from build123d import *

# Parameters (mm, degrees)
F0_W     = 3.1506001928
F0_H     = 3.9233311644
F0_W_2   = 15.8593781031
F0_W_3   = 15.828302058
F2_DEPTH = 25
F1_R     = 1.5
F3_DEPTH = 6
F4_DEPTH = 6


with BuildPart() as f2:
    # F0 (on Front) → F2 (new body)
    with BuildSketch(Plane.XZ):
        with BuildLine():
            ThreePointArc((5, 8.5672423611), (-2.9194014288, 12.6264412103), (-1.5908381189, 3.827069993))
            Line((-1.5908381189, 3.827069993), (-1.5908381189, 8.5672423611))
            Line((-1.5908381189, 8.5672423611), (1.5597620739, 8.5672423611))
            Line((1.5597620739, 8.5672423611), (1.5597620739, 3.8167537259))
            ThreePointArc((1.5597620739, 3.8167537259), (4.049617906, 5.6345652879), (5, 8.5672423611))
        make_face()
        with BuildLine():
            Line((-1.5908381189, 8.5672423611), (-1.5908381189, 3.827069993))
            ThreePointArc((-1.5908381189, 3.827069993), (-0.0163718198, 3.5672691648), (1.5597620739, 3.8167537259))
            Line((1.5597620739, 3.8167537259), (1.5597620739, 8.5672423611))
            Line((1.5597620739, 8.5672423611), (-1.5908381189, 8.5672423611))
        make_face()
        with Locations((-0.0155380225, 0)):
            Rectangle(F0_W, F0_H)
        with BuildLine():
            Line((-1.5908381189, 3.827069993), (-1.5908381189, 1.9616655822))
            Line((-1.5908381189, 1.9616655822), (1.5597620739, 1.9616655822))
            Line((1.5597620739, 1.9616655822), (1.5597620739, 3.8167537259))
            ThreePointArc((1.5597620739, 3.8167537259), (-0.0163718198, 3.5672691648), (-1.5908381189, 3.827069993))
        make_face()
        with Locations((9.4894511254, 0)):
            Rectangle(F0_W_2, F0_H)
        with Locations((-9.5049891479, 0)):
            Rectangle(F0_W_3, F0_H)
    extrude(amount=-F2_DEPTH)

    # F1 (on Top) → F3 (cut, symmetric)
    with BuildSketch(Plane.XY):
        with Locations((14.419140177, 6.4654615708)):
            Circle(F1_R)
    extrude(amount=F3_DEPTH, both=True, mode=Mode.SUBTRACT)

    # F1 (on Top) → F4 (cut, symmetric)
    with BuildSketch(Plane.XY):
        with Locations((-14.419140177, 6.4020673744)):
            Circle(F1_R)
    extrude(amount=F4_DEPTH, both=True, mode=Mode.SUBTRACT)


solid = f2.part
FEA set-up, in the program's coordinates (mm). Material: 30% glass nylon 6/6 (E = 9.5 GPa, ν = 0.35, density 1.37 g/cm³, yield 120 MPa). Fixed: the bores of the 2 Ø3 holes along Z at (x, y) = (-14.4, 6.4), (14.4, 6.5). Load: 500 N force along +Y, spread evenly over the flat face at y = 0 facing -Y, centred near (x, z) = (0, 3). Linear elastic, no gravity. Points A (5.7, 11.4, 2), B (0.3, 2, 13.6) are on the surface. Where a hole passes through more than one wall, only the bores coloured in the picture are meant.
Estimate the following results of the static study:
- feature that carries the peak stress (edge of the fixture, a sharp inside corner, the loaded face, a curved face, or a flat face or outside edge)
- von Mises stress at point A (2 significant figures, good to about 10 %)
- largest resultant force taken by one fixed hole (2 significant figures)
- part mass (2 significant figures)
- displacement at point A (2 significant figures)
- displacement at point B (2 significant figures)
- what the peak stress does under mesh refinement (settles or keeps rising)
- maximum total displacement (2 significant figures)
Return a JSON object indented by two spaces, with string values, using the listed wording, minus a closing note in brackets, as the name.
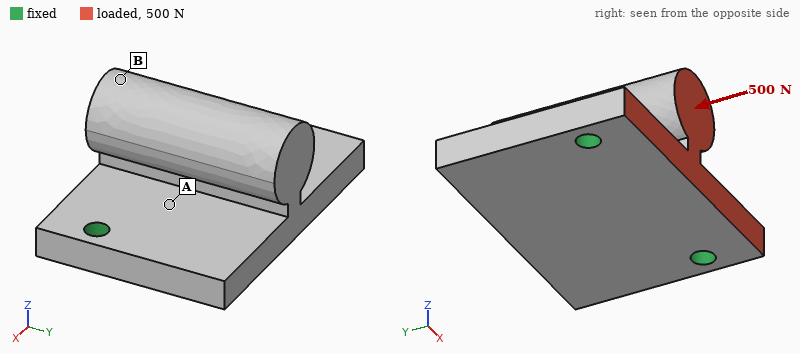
{
  "feature that carries the peak stress": "edge of the fixture",
  "von Mises stress at point A": "9.7 MPa",
  "largest resultant force taken by one fixed hole": "250 N",
  "part mass": "7.5 g",
  "displacement at point A": "0.034 mm",
  "displacement at point B": "0.13 mm",
  "what the peak stress does under mesh refinement": "keeps rising",
  "maximum total displacement": "0.18 mm"
}
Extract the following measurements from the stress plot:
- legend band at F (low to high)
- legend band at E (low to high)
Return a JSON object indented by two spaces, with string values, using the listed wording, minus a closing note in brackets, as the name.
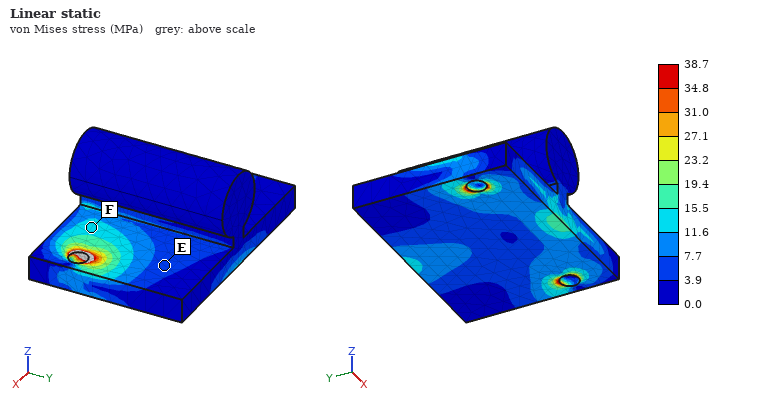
{
  "legend band at F": "11.6 to 15.5 MPa",
  "legend band at E": "3.9 to 7.7 MPa"
}
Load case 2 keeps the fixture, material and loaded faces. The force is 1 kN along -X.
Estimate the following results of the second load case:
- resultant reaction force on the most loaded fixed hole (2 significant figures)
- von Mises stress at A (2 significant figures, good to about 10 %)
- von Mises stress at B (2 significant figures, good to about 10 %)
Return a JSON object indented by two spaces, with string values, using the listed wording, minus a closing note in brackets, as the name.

{
  "resultant reaction force on the most loaded fixed hole": "560 N",
  "von Mises stress at A": "14 MPa",
  "von Mises stress at B": "8.7 MPa"
}
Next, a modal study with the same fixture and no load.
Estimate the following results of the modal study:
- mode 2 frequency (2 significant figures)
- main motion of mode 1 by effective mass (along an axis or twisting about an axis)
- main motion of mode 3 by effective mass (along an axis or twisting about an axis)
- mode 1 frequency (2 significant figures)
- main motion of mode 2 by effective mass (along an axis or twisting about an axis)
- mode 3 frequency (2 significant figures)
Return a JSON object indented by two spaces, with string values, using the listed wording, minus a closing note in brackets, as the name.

{
  "mode 2 frequency": "4500 Hz",
  "main motion of mode 1 by effective mass": "along Z",
  "main motion of mode 3 by effective mass": "along Z",
  "mode 1 frequency": "2600 Hz",
  "main motion of mode 2 by effective mass": "along X",
  "mode 3 frequency": "6200 Hz"
}
